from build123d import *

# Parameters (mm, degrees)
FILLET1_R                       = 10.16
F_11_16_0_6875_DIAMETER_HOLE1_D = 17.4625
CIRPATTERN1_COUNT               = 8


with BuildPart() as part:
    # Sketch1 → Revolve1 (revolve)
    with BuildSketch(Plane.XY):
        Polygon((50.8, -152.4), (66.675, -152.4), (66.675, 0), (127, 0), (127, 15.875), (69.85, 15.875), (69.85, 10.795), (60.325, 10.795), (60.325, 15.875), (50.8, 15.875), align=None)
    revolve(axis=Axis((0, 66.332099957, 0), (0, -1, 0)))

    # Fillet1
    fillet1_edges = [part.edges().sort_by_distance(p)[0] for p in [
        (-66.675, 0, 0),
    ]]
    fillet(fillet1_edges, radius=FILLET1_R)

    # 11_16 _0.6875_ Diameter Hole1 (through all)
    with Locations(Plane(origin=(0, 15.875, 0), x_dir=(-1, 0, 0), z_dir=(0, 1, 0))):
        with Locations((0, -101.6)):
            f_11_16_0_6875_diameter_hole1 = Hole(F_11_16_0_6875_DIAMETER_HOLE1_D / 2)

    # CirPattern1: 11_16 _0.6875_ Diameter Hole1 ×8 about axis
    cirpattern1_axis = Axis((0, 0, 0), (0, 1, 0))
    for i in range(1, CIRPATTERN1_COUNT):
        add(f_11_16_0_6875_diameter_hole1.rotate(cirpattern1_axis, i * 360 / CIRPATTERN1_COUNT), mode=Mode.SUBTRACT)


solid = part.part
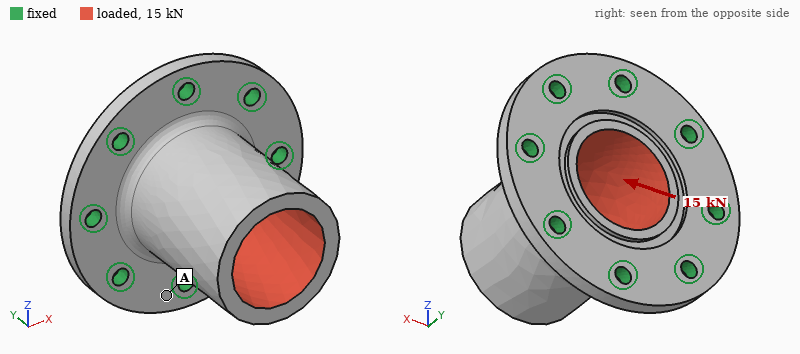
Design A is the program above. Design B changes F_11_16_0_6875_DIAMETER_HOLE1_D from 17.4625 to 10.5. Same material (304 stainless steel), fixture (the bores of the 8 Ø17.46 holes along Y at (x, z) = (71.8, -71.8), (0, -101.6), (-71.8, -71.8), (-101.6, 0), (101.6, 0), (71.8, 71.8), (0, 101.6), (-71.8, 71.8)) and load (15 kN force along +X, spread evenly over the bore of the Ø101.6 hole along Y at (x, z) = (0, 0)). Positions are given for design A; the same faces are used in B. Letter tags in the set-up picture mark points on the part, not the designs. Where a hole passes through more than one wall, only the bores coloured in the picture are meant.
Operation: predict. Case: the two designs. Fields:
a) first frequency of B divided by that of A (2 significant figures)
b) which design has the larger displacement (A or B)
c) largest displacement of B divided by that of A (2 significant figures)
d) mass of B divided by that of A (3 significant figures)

0.91
B
1.2
1.01
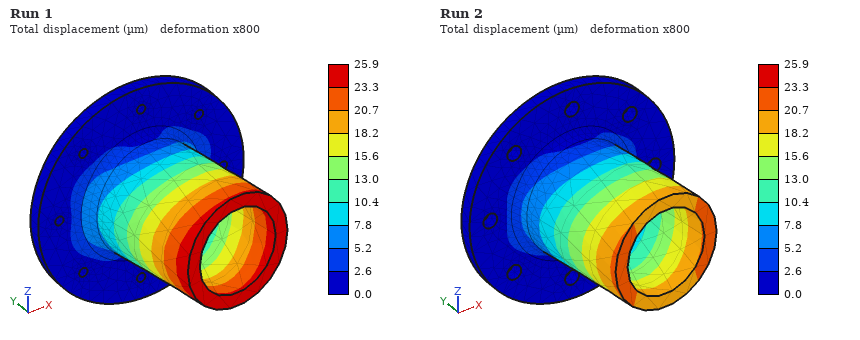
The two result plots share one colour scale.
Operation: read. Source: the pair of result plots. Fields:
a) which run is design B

Run 1
